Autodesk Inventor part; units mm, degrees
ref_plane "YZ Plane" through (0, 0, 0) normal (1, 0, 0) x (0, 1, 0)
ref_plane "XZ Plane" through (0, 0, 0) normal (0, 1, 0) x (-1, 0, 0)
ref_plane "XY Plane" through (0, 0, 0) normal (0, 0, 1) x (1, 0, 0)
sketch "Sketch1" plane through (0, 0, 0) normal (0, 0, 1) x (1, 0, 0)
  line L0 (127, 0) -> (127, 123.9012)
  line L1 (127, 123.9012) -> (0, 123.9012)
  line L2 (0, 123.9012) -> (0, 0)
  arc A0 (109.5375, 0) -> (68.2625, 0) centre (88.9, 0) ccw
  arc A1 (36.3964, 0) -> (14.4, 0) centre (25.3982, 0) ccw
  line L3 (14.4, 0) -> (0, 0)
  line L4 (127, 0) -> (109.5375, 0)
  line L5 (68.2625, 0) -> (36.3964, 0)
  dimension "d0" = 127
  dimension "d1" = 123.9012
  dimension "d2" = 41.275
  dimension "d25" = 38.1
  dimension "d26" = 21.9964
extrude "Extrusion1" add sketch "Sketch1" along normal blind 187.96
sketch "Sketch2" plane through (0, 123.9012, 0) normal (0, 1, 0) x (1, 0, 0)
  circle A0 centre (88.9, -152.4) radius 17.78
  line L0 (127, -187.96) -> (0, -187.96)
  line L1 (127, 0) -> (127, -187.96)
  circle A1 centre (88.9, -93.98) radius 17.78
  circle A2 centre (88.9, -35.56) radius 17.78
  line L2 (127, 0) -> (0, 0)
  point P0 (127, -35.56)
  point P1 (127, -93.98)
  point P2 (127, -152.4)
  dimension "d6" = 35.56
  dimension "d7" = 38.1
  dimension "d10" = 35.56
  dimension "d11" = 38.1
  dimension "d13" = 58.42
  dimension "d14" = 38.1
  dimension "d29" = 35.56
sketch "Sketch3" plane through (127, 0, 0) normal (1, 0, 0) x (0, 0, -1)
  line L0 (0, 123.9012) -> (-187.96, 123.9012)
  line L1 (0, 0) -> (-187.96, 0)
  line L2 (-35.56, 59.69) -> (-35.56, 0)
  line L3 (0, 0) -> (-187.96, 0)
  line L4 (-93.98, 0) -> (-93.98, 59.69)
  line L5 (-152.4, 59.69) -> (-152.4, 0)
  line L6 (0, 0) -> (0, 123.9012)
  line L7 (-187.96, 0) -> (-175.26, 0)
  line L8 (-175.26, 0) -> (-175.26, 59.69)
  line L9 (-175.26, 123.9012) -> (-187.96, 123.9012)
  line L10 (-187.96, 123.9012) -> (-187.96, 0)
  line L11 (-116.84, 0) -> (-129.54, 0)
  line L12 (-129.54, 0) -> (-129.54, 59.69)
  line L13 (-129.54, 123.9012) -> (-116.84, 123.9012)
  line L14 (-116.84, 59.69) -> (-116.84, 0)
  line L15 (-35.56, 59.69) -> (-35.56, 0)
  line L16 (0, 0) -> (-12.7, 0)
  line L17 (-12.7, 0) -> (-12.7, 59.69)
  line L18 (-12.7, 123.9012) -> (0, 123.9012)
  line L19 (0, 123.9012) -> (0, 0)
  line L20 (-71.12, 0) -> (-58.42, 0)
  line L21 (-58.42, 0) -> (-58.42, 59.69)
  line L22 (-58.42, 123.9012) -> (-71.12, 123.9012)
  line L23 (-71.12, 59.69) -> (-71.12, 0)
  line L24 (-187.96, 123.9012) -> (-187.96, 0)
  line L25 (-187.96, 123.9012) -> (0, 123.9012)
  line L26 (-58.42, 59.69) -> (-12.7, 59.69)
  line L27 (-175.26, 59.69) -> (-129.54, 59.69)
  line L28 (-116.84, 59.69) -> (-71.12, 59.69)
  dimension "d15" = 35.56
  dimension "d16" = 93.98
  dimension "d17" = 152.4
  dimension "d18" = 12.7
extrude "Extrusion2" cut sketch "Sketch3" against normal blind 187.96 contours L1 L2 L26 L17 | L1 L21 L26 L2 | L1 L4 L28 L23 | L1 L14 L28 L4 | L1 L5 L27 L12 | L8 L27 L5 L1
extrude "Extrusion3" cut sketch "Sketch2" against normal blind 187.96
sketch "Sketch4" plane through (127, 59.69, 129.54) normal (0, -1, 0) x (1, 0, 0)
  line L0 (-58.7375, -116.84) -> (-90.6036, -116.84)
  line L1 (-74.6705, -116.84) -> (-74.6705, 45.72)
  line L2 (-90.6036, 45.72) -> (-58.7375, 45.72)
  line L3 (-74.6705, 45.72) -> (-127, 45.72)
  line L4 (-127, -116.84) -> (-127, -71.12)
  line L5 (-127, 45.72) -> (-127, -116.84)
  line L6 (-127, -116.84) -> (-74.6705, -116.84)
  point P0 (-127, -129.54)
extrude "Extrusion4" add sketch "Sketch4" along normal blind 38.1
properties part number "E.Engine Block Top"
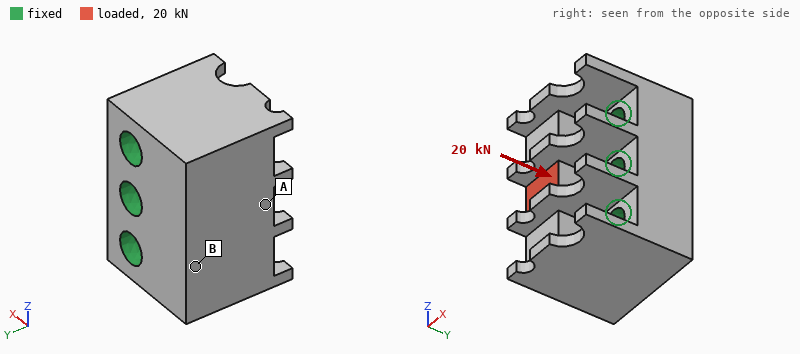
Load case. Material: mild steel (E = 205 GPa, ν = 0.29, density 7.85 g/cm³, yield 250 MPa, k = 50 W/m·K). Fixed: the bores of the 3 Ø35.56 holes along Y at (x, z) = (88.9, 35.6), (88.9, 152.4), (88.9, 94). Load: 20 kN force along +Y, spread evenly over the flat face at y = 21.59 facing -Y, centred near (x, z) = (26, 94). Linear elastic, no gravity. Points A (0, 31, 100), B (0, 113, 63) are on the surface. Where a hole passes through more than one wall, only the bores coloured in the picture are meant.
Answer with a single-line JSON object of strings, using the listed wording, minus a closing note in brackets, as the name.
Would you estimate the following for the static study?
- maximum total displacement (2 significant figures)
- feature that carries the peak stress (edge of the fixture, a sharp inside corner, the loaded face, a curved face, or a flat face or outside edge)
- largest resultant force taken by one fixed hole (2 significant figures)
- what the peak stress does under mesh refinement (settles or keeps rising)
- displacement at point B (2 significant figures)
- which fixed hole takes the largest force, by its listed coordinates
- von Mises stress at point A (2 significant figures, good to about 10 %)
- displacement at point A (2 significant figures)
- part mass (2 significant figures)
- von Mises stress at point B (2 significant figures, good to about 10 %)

{"maximum total displacement": "5.6 µm", "feature that carries the peak stress": "edge of the fixture", "largest resultant force taken by one fixed hole": "8.4 kN", "what the peak stress does under mesh refinement": "keeps rising", "displacement at point B": "2.8 µm", "which fixed hole takes the largest force, by its listed coordinates": "(88.9, 94)", "von Mises stress at point A": "7.6 MPa", "displacement at point A": "5.1 µm", "part mass": "15 kg", "von Mises stress at point B": "1.7 MPa"}
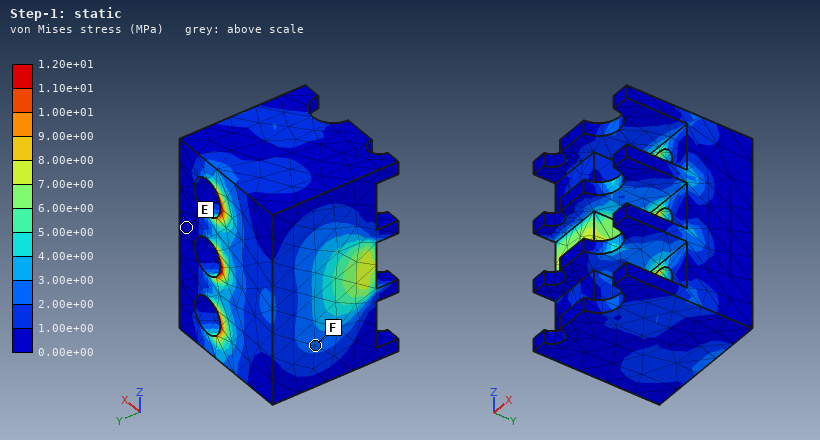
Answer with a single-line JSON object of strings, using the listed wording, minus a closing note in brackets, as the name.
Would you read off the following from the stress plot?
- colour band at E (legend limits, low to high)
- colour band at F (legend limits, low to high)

{"colour band at E": "0.00e+00 to 1.00e+00 MPa", "colour band at F": "2.00e+00 to 3.00e+00 MPa"}
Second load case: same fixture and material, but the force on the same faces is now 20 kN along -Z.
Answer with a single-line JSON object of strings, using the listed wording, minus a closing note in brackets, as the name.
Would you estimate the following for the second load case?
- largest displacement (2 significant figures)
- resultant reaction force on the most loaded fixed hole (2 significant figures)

{"largest displacement": "5.1 µm", "resultant reaction force on the most loaded fixed hole": "13 kN"}
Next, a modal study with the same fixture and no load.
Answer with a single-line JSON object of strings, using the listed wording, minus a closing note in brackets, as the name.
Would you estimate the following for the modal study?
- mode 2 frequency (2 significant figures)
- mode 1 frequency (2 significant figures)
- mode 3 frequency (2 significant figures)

{"mode 2 frequency": "3700 Hz", "mode 1 frequency": "3700 Hz", "mode 3 frequency": "4000 Hz"}
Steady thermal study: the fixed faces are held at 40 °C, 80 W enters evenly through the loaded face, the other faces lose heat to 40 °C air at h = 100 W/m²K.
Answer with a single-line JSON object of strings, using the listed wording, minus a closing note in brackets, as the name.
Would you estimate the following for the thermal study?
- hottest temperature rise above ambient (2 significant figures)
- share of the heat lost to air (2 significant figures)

{"hottest temperature rise above ambient": "21 K", "share of the heat lost to air": "41 %"}
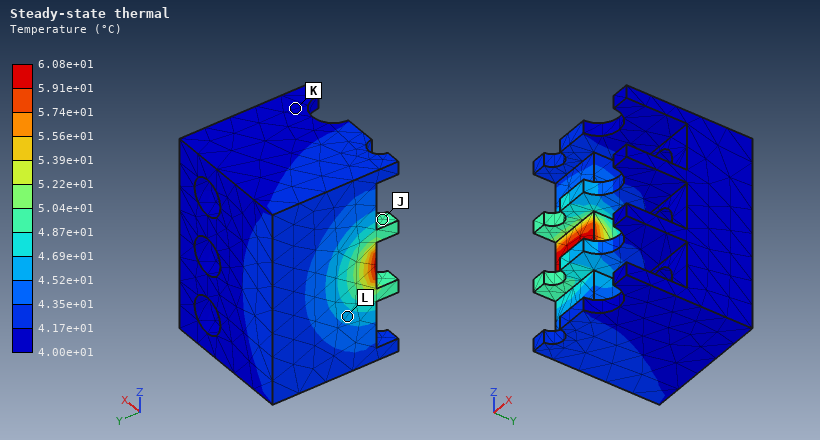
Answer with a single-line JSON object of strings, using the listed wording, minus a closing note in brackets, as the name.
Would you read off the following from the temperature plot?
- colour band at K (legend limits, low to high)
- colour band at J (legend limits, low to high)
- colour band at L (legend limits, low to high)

{"colour band at K": "4.00e+01 to 4.17e+01 °C", "colour band at J": "4.87e+01 to 5.04e+01 °C", "colour band at L": "4.52e+01 to 4.69e+01 °C"}
